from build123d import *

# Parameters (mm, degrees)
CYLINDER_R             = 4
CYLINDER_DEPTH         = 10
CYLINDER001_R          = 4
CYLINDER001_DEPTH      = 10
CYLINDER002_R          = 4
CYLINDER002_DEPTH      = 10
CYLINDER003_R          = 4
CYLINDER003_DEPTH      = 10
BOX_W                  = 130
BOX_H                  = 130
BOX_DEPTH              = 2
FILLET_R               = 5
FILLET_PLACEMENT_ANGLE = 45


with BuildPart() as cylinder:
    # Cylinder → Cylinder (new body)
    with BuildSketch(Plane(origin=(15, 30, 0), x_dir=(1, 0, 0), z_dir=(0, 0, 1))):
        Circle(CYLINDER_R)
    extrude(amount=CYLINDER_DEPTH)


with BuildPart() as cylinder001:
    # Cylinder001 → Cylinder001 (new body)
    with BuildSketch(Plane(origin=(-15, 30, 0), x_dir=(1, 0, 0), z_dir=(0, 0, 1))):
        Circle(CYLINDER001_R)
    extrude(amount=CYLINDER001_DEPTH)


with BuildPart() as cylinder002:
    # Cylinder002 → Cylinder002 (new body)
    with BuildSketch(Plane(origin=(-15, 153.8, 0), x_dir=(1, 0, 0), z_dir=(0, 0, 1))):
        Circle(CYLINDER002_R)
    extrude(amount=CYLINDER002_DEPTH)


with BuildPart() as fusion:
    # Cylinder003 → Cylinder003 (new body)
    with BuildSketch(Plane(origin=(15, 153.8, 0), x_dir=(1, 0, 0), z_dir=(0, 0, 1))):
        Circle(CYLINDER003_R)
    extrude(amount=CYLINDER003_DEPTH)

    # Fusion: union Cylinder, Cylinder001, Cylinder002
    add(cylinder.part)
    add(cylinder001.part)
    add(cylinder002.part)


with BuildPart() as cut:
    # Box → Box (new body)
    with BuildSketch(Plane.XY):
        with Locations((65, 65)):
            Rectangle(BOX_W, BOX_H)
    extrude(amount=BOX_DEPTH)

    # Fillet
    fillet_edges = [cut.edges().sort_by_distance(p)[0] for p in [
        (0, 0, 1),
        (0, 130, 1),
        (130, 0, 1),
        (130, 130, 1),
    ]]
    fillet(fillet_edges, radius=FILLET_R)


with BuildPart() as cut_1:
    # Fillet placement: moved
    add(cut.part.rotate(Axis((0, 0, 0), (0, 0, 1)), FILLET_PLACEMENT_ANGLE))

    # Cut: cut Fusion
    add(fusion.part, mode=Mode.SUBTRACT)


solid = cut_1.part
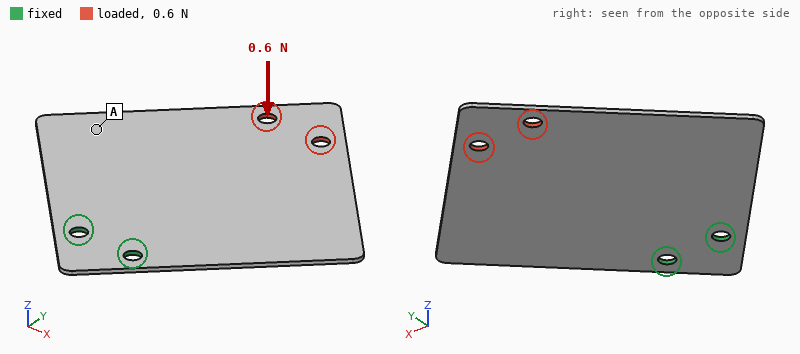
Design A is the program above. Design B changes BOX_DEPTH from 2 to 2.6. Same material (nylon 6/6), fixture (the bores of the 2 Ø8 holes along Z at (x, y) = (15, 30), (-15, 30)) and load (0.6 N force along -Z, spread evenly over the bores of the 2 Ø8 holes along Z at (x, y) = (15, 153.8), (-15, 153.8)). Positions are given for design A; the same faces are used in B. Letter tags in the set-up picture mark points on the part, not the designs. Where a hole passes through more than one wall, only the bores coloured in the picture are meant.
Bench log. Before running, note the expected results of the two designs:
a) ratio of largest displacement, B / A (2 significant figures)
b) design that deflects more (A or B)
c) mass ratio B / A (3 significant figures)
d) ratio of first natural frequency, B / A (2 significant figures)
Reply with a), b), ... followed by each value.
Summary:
a) 0.46
b) A
c) 1.30
d) 1.3
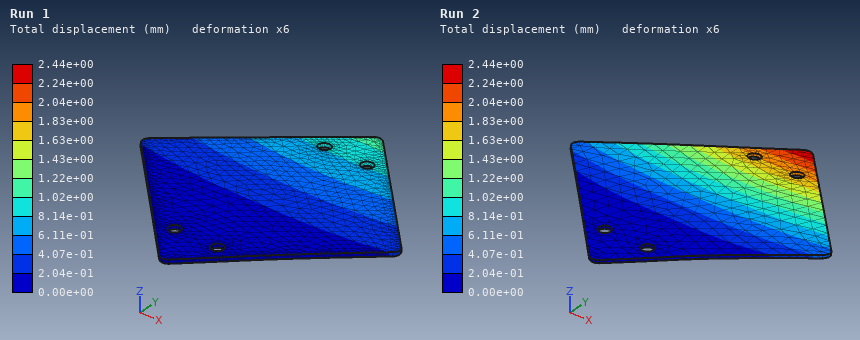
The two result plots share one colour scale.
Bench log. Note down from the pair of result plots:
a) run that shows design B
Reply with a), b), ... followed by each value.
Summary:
a) Run 1
